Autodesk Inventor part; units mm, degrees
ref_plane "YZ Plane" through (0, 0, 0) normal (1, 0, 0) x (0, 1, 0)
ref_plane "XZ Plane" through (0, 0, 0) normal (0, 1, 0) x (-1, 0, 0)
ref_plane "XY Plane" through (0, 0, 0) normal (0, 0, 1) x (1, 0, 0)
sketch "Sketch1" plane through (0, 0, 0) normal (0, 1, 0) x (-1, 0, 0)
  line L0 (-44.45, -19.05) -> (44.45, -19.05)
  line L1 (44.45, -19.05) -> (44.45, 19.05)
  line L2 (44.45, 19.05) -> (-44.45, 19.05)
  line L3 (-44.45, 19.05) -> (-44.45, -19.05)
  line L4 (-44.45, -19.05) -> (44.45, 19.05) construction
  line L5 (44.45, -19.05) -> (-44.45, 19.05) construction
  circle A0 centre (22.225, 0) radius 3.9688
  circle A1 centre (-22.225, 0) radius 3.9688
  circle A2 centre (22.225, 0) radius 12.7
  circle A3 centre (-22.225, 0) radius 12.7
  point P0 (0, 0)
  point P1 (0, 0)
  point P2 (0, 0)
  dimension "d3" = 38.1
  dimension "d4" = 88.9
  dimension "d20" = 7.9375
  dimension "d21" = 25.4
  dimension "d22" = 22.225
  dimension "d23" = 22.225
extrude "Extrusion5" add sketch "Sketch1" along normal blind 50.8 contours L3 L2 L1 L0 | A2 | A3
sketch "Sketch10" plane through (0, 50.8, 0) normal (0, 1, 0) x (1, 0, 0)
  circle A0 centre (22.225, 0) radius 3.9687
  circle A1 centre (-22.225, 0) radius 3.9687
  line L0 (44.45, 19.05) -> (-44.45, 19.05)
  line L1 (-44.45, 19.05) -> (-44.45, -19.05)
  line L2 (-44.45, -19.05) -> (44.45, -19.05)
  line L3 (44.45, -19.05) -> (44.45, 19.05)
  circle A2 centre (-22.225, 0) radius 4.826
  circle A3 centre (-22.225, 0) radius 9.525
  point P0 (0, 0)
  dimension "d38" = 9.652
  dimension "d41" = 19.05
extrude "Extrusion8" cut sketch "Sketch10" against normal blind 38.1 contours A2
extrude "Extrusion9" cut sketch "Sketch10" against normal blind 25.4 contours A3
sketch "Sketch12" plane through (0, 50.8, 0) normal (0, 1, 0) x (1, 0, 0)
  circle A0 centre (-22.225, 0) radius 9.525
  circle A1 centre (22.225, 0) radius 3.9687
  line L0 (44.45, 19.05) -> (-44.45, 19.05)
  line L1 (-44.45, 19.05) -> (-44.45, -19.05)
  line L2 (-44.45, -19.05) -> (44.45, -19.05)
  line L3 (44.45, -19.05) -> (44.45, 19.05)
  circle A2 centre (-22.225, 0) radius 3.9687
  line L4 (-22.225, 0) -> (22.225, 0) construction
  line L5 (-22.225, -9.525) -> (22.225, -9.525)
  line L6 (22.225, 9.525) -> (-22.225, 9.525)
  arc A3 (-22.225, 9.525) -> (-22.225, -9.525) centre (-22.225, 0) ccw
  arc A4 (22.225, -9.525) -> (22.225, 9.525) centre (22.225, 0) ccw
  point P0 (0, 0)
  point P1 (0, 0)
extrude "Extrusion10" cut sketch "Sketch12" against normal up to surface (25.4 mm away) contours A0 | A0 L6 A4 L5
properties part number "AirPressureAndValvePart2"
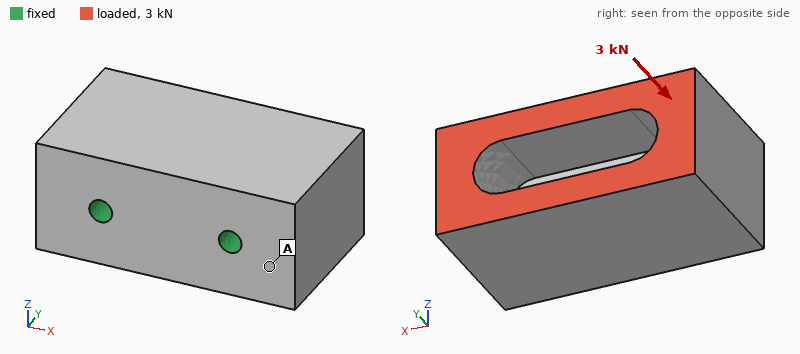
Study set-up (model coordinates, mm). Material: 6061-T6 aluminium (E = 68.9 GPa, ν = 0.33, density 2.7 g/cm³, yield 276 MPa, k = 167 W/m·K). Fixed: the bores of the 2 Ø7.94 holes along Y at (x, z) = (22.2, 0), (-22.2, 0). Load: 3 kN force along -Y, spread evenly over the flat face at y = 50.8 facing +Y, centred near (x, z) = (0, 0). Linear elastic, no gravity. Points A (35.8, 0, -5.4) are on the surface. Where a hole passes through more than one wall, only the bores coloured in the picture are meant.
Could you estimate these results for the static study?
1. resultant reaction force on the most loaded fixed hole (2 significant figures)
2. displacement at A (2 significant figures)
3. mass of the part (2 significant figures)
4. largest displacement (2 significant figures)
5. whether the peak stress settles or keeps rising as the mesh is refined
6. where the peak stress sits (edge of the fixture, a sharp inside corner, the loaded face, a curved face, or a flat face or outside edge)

1.5 kN
0.62 µm
380 g
2.2 µm
keeps rising
edge of the fixture
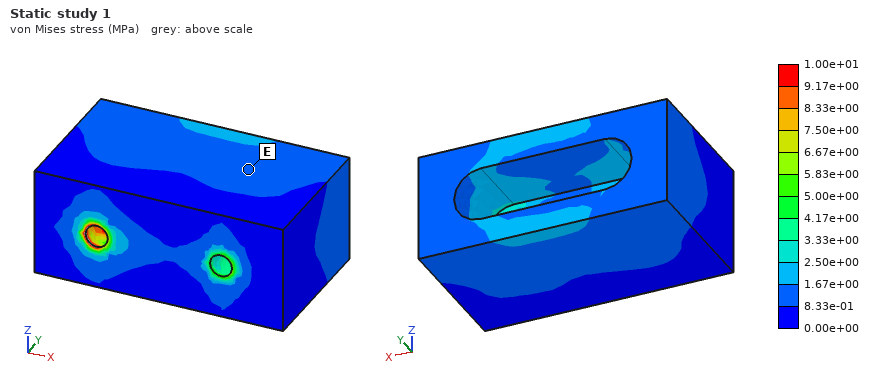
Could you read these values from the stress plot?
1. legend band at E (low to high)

8.33e-01 to 1.67e+00 MPa
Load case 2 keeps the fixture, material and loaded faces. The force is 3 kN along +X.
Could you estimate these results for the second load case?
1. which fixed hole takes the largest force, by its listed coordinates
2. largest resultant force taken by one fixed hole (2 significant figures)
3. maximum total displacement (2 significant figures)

(22.2, 0)
3.0 kN
8.5 µm
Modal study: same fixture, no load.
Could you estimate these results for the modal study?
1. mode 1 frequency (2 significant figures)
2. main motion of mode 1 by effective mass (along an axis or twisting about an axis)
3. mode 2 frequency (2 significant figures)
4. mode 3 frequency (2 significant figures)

5600 Hz
along Z
9600 Hz
9900 Hz
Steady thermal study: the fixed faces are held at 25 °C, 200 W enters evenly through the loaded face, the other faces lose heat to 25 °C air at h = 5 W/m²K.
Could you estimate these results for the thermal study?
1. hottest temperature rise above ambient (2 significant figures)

26 K
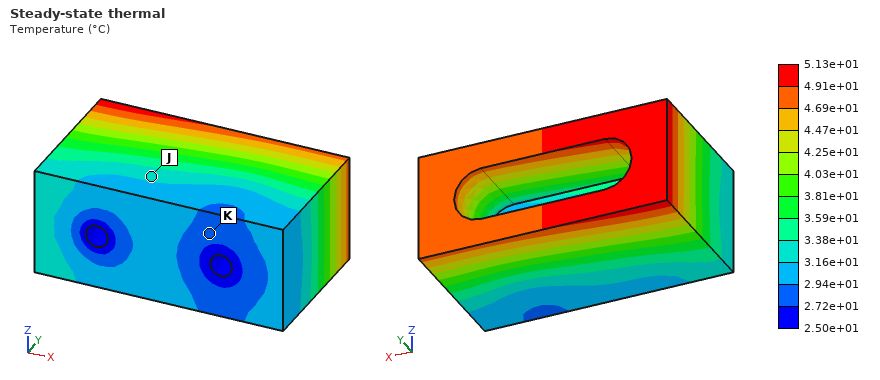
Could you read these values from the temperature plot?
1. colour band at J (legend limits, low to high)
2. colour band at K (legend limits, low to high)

3.16e+01 to 3.38e+01 °C
2.72e+01 to 2.94e+01 °C
